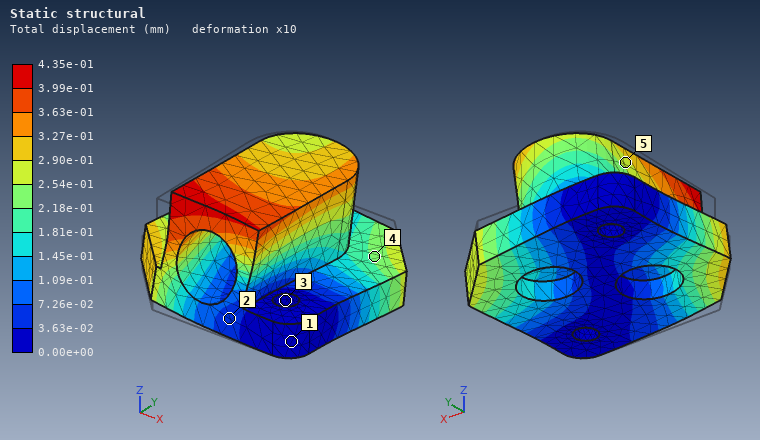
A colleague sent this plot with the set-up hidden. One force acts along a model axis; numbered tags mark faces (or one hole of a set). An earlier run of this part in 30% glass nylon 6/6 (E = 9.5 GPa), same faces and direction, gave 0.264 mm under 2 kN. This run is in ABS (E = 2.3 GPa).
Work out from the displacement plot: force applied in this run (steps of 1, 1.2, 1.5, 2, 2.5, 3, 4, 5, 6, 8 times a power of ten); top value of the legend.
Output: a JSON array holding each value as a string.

["800 N", "4.35e-01 mm"]
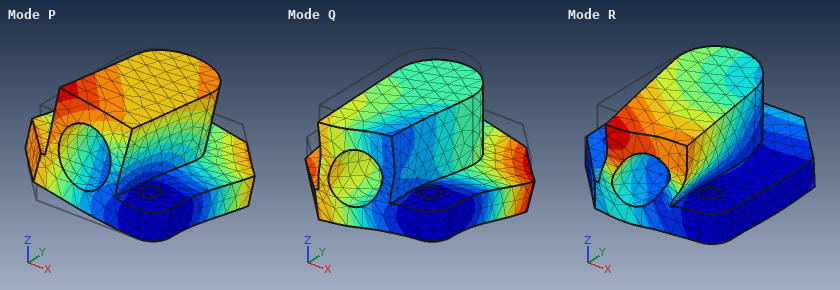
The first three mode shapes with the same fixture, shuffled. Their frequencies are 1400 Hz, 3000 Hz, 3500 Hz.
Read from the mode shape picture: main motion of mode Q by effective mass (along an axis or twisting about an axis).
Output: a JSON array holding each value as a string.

["along Z"]
